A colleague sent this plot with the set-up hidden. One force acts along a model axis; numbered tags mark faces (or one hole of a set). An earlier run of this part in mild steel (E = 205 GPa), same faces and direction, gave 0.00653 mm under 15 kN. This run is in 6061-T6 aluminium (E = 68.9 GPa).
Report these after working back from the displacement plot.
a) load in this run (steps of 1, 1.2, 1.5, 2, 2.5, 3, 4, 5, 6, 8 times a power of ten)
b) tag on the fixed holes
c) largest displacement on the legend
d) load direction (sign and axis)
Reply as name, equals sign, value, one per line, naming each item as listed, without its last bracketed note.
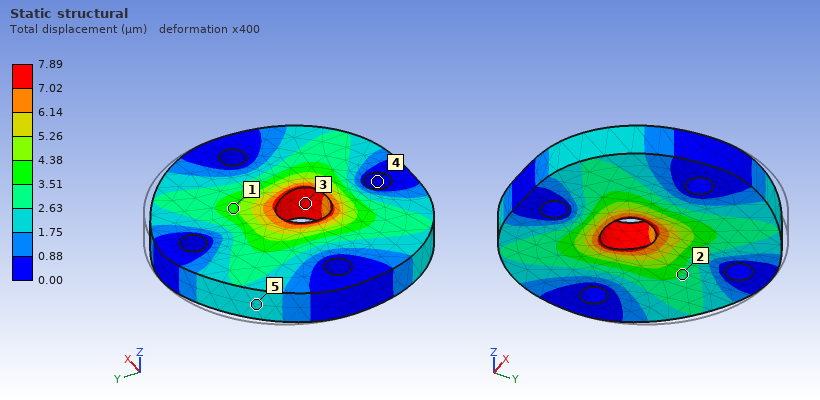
load in this run = 6 kN
tag on the fixed holes = 4
largest displacement on the legend = 7.89 µm
load direction = -Y
